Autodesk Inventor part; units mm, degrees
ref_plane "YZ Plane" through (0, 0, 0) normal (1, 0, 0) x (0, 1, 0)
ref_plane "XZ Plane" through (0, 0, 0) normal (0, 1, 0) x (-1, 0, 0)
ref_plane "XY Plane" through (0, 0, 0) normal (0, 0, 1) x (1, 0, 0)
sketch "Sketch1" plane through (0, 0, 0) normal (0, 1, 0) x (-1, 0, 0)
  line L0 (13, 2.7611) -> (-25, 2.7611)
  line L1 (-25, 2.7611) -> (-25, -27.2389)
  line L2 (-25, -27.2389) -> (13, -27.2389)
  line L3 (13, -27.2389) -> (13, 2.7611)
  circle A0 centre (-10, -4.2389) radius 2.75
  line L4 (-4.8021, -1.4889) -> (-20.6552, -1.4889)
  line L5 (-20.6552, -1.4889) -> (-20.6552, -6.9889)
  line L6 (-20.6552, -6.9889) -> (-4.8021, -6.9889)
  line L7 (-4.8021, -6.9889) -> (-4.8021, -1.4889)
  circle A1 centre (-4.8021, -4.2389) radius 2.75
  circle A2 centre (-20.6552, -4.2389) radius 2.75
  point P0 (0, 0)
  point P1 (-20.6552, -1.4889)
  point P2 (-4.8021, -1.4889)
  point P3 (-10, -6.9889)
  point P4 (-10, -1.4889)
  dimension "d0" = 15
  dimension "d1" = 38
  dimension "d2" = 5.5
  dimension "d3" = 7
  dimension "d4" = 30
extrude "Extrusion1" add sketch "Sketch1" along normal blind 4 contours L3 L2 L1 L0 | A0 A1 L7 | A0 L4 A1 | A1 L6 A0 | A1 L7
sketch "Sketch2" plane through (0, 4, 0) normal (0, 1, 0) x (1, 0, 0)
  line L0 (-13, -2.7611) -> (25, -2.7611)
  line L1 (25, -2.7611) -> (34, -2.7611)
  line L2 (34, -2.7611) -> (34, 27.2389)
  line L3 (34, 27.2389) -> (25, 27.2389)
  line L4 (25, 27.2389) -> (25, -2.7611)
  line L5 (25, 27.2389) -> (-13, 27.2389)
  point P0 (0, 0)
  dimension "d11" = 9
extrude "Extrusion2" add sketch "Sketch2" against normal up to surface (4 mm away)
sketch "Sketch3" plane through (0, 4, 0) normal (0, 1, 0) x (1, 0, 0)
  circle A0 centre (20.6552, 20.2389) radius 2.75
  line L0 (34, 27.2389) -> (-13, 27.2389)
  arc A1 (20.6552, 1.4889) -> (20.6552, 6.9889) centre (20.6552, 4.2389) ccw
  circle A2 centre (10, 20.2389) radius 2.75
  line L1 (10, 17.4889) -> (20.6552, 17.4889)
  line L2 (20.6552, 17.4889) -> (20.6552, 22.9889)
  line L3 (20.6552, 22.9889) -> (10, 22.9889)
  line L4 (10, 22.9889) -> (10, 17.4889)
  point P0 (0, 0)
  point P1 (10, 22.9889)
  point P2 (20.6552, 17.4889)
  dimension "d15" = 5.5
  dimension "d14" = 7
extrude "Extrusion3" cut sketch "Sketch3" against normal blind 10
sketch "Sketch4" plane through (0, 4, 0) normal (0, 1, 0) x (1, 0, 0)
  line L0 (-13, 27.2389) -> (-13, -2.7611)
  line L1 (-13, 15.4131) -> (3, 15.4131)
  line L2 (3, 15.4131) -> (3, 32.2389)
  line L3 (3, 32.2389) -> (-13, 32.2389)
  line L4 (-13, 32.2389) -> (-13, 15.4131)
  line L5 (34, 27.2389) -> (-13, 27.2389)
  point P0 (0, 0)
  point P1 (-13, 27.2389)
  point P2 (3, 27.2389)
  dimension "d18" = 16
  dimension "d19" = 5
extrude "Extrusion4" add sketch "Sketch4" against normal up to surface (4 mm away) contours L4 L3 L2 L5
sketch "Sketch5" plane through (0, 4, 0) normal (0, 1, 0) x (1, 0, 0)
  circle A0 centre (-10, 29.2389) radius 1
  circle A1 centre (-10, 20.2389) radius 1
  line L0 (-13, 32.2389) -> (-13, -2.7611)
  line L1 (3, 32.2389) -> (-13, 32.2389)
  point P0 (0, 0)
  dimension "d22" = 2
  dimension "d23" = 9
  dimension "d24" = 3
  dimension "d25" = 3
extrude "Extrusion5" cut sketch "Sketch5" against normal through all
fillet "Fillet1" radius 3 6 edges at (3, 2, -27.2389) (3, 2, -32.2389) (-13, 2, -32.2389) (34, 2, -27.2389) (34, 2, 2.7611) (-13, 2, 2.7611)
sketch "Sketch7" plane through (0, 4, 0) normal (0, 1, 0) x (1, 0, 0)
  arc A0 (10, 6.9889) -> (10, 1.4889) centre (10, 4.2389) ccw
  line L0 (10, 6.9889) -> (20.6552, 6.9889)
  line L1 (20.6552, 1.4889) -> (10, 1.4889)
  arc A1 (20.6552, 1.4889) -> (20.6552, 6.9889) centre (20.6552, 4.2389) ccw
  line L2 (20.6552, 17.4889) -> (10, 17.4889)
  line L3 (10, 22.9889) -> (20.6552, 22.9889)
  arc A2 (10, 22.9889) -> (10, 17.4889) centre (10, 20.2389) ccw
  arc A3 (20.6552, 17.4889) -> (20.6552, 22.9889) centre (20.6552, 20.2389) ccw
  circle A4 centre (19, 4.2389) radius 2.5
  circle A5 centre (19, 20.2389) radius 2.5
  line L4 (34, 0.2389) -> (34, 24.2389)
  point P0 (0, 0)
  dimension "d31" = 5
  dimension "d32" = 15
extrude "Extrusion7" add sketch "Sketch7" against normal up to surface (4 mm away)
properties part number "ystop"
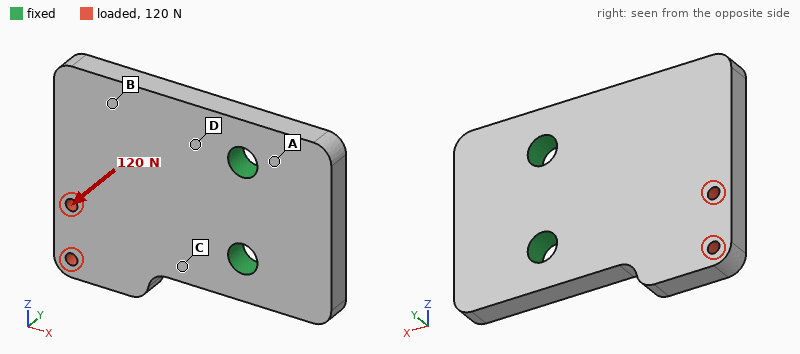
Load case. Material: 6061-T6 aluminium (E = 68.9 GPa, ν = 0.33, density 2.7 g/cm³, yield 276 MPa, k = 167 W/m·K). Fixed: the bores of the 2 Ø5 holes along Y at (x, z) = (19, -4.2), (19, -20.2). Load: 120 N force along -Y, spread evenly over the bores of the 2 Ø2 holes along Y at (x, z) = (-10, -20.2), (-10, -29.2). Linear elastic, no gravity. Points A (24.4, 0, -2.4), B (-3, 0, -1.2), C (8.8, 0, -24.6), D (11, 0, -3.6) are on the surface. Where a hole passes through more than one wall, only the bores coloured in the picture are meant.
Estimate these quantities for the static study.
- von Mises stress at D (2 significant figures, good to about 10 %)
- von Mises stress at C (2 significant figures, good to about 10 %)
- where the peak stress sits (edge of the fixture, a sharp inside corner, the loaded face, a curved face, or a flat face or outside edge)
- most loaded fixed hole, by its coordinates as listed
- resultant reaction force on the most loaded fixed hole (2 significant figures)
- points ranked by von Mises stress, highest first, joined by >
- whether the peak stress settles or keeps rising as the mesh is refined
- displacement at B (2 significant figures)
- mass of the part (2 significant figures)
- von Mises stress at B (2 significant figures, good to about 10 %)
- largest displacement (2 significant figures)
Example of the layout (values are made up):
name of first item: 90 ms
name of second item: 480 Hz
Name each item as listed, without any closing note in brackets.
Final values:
von Mises stress at D: 26 MPa
von Mises stress at C: 36 MPa
where the peak stress sits: edge of the fixture
most loaded fixed hole, by its coordinates as listed: (19, -20.2)
resultant reaction force on the most loaded fixed hole: 130 N
points ranked by von Mises stress, highest first, joined by >: C > D > B > A
whether the peak stress settles or keeps rising as the mesh is refined: keeps rising
displacement at B: 0.033 mm
mass of the part: 16 g
von Mises stress at B: 13 MPa
largest displacement: 0.12 mm
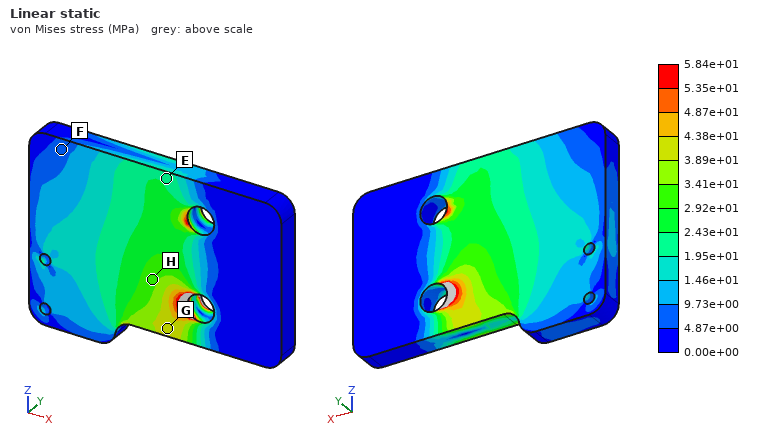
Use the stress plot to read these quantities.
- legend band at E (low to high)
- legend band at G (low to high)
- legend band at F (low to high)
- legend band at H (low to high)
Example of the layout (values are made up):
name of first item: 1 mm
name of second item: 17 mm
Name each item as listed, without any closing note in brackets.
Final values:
legend band at E: 1.95e+01 to 2.43e+01 MPa
legend band at G: 3.89e+01 to 4.38e+01 MPa
legend band at F: 4.87e+00 to 9.73e+00 MPa
legend band at H: 2.92e+01 to 3.41e+01 MPa
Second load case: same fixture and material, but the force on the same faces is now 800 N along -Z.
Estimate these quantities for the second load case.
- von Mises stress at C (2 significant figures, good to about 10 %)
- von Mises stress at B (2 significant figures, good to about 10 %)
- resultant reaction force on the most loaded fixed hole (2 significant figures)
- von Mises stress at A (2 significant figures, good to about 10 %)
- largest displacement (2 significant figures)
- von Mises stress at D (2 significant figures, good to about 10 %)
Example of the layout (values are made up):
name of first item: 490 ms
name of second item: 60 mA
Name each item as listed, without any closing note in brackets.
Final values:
von Mises stress at C: 21 MPa
von Mises stress at B: 8.7 MPa
resultant reaction force on the most loaded fixed hole: 1.3 kN
von Mises stress at A: 7.0 MPa
largest displacement: 29 µm
von Mises stress at D: 23 MPa
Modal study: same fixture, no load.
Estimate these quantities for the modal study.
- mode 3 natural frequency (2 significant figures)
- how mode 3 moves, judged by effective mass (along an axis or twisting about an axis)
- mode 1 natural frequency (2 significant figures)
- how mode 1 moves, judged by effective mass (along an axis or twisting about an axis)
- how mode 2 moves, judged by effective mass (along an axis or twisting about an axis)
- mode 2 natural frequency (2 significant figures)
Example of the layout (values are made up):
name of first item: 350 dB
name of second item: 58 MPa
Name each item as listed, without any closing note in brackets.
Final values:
mode 3 natural frequency: 14 kHz
how mode 3 moves, judged by effective mass: along Z
mode 1 natural frequency: 3300 Hz
how mode 1 moves, judged by effective mass: along Y
how mode 2 moves, judged by effective mass: twisting about X
mode 2 natural frequency: 6700 Hz
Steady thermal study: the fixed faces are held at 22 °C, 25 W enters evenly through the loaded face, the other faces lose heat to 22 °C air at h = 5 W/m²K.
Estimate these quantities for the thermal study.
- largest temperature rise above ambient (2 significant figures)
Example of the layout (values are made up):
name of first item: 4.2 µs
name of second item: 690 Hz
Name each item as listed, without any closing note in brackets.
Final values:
largest temperature rise above ambient: 53 K
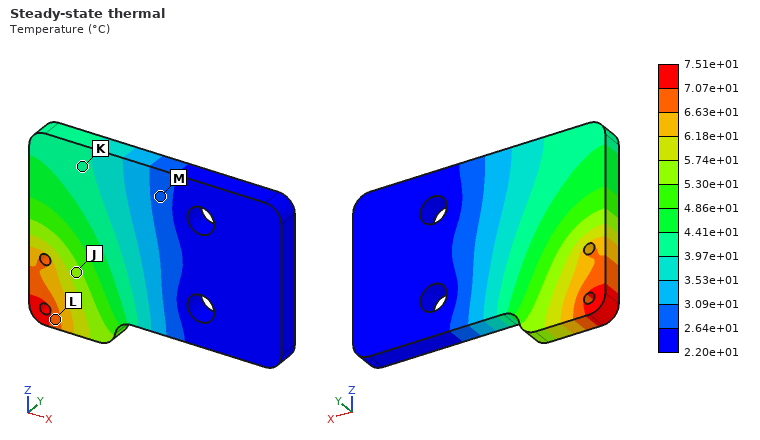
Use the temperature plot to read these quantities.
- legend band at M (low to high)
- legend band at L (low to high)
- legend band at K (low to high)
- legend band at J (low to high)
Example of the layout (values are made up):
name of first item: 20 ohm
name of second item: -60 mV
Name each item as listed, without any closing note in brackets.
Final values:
legend band at M: 2.64e+01 to 3.09e+01 °C
legend band at L: 6.63e+01 to 7.07e+01 °C
legend band at K: 3.97e+01 to 4.41e+01 °C
legend band at J: 5.30e+01 to 5.74e+01 °C
